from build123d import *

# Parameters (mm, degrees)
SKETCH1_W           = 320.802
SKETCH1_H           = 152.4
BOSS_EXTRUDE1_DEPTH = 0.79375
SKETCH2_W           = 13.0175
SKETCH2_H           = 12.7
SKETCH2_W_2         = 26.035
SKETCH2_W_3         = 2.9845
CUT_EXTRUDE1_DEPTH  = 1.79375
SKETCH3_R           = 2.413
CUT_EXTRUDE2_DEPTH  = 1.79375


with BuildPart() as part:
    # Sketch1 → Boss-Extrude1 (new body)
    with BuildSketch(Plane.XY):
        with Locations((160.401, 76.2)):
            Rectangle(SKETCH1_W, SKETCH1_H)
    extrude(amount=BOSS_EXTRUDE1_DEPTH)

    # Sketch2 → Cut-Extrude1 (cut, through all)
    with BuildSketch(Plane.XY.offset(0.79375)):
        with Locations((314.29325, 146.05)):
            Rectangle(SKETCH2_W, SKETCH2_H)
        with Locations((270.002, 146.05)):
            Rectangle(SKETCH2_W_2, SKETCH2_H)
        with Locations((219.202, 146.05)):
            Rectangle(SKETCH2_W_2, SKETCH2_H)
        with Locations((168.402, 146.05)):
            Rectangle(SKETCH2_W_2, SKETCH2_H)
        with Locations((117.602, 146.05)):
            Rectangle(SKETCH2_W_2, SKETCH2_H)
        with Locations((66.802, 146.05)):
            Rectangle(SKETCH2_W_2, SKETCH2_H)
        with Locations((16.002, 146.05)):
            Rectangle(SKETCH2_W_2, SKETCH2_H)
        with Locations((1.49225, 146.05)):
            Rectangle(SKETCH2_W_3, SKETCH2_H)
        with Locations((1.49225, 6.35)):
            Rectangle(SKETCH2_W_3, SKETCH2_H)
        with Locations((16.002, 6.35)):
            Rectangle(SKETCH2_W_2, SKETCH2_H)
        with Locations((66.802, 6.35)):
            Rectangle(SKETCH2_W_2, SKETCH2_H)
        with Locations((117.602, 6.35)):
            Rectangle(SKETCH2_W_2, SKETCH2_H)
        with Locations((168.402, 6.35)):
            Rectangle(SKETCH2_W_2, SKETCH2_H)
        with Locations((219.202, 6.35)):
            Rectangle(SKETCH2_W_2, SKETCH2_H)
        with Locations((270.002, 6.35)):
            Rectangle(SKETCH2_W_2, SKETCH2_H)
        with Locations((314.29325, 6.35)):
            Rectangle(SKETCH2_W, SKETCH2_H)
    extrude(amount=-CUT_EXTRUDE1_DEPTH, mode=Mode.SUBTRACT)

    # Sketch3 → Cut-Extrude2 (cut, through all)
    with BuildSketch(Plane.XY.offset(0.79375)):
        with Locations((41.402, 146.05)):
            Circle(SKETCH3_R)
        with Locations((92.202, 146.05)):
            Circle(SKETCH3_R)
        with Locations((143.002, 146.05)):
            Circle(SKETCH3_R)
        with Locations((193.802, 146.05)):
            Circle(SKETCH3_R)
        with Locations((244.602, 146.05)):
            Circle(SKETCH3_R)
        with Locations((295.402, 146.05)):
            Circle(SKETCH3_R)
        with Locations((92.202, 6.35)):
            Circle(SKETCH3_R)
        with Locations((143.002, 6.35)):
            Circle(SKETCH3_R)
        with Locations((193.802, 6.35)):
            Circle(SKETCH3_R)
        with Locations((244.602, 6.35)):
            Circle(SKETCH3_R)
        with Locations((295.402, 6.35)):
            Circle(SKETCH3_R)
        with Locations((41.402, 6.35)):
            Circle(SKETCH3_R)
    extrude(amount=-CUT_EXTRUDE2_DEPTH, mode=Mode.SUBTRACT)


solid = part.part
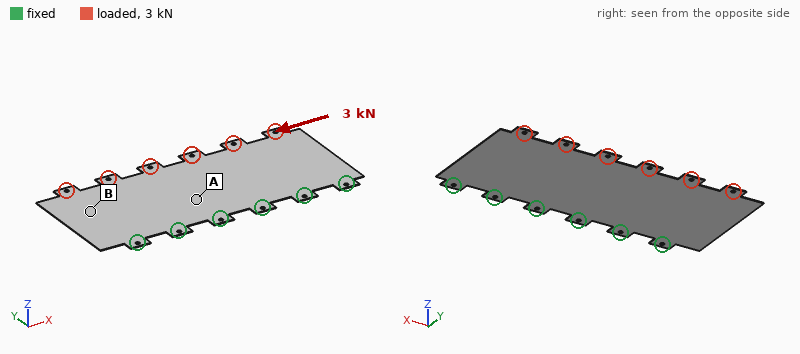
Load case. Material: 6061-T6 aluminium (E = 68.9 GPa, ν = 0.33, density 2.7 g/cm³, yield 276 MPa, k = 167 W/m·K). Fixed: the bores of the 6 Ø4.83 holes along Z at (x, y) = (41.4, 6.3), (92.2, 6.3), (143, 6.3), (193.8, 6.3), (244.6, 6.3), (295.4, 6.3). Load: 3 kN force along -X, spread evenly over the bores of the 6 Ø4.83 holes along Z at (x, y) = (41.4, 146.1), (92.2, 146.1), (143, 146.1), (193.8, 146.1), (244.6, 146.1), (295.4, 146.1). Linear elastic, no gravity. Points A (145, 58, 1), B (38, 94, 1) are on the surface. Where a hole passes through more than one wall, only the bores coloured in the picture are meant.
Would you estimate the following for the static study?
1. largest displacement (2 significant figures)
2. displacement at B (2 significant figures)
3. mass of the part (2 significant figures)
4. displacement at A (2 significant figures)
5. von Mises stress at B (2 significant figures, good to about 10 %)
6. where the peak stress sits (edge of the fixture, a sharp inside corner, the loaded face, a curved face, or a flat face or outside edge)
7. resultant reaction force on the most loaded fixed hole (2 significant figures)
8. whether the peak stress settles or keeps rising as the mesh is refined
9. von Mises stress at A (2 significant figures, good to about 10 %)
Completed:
0.19 mm
0.098 mm
95 g
0.051 mm
12 MPa
edge of the fixture
1.4 kN
keeps rising
31 MPa
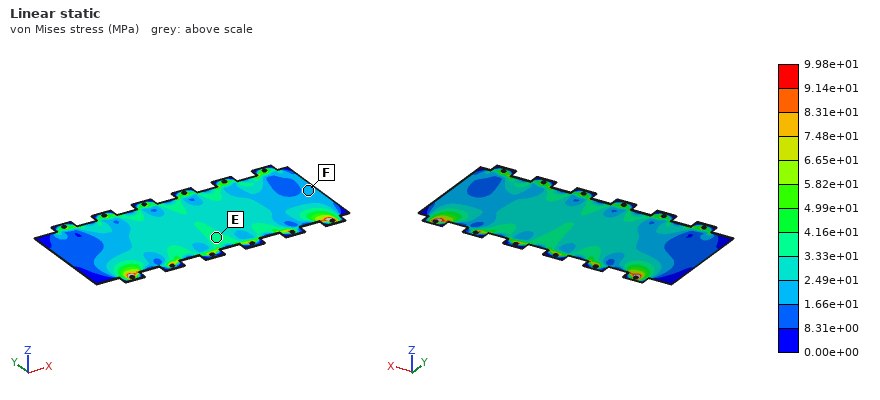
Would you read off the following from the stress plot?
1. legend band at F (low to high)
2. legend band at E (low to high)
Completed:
1.66e+01 to 2.49e+01 MPa
3.33e+01 to 4.16e+01 MPa
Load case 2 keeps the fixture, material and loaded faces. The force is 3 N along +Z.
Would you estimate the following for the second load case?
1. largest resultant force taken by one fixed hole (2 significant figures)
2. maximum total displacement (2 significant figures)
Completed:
0.71 N
3.7 mm
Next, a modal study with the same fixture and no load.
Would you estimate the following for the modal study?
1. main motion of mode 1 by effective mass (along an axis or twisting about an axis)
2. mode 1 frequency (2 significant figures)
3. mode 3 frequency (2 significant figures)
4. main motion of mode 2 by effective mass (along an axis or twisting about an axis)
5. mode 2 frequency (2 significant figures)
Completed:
along Z
30 Hz
79 Hz
twisting about Y
44 Hz
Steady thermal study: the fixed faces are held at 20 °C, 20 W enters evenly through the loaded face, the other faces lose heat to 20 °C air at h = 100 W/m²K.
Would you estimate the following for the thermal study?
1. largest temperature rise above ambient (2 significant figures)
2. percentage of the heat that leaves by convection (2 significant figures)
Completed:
21 K
100 %
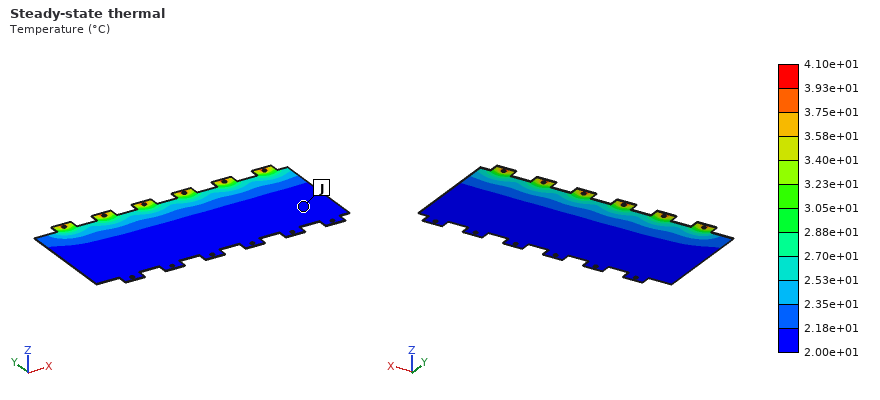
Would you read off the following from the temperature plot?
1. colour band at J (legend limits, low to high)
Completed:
2.00e+01 to 2.18e+01 °C
